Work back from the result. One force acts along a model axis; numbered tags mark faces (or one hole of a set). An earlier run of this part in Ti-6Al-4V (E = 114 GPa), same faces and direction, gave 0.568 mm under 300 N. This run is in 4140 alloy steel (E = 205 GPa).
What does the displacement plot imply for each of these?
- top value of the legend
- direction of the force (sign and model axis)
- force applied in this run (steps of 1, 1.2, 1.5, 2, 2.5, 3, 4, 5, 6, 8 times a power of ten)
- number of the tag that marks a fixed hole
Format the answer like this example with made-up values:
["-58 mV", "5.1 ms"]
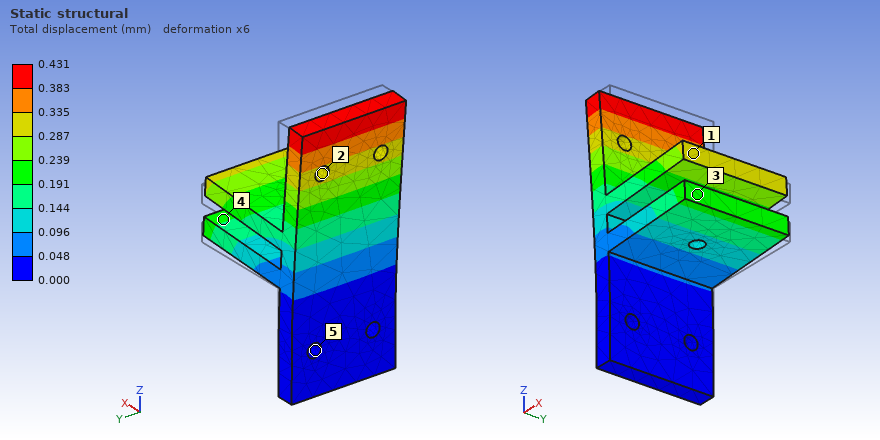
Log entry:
["0.431 mm", "-X", "400 N", "5"]
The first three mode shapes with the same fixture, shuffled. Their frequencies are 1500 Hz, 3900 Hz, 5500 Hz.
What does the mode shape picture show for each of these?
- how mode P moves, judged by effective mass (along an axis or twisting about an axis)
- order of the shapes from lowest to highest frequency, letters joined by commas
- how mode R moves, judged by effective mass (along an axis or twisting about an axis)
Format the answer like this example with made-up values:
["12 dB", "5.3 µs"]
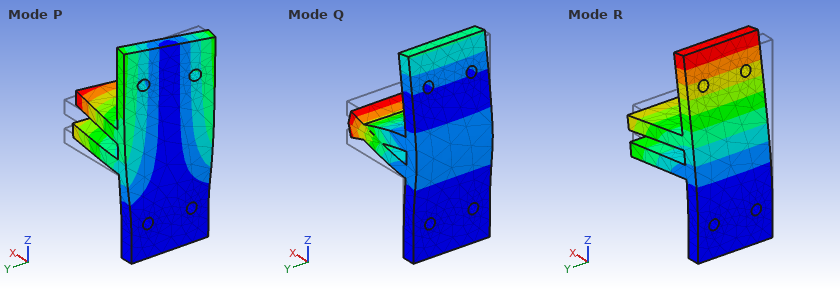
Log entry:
["along Y", "R, P, Q", "along X"]
